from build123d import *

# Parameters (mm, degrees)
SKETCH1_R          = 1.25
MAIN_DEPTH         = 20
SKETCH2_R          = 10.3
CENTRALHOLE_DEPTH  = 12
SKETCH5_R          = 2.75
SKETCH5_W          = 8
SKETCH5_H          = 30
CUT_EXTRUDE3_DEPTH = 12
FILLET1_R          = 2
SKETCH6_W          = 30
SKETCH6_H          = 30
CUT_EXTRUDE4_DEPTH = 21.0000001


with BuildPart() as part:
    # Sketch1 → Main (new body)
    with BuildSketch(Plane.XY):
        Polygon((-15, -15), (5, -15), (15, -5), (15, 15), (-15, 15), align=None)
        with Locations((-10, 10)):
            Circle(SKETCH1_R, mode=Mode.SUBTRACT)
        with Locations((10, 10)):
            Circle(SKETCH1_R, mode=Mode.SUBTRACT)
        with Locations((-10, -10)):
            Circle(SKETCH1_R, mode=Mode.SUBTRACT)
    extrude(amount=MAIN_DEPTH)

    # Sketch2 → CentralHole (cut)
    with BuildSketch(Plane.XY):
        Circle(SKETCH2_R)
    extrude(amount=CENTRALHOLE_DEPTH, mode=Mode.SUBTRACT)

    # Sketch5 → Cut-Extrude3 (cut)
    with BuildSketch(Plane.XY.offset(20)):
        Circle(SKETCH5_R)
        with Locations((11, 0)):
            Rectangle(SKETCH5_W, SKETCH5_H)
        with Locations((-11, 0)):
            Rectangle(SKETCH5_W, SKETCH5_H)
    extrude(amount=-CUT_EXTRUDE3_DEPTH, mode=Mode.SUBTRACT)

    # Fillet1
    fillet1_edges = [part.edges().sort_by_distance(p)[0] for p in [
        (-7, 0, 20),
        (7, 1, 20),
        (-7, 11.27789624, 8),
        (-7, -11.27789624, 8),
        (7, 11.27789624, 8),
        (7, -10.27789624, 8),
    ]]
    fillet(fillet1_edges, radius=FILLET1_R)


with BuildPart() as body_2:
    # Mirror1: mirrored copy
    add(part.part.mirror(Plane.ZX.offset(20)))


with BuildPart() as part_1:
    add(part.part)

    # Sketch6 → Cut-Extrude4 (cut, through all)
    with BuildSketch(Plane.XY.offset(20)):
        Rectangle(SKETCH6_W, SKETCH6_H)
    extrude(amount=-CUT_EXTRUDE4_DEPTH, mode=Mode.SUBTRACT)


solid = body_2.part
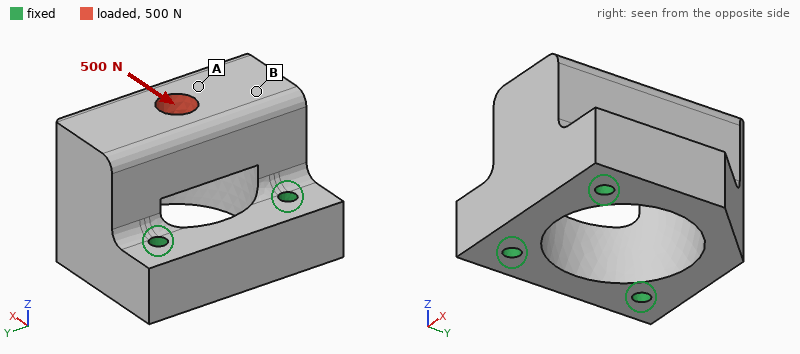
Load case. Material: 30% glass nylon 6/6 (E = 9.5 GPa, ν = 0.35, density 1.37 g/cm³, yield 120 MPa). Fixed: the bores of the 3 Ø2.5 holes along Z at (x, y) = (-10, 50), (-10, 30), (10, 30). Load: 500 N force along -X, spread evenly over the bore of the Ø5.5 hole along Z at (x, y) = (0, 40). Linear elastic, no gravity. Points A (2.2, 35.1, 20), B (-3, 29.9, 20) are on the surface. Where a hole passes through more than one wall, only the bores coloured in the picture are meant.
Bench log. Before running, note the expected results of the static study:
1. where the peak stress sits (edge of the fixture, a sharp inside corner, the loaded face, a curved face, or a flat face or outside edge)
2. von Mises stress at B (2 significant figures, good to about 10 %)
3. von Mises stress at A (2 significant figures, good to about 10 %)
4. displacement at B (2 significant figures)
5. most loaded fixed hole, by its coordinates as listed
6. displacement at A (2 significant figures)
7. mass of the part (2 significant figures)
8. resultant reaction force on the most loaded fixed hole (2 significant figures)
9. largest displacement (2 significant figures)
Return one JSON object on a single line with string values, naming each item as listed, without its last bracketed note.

{"where the peak stress sits": "edge of the fixture", "von Mises stress at B": "4.1 MPa", "von Mises stress at A": "8.5 MPa", "displacement at B": "32 µm", "most loaded fixed hole, by its coordinates as listed": "(10, 30)", "displacement at A": "42 µm", "mass of the part": "11 g", "resultant reaction force on the most loaded fixed hole": "290 N", "largest displacement": "59 µm"}
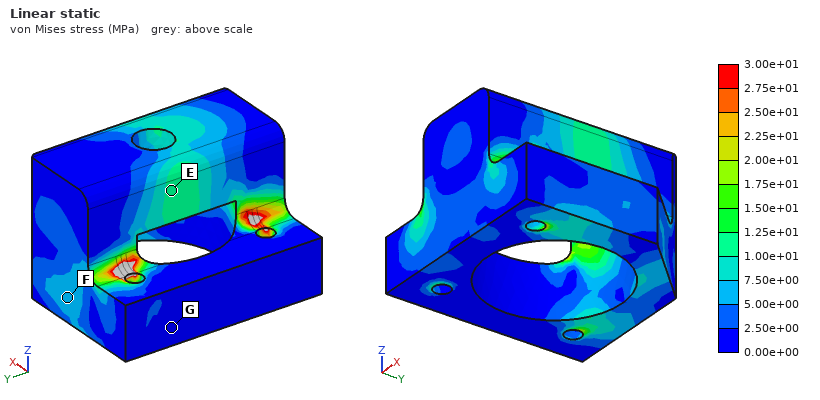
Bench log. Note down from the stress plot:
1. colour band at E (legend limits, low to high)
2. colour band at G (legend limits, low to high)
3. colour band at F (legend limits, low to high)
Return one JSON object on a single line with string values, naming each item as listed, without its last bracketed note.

{"colour band at E": "1.00e+01 to 1.25e+01 MPa", "colour band at G": "0.00e+00 to 2.50e+00 MPa", "colour band at F": "5.00e+00 to 7.50e+00 MPa"}
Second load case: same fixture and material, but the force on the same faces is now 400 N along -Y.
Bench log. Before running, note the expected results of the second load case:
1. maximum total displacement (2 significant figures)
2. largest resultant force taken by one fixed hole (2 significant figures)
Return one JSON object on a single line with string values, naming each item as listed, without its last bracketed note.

{"maximum total displacement": "42 µm", "largest resultant force taken by one fixed hole": "170 N"}
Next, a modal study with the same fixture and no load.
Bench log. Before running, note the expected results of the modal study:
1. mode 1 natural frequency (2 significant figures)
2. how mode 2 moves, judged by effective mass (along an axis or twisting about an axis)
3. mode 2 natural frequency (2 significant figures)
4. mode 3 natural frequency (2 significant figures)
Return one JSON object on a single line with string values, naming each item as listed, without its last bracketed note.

{"mode 1 natural frequency": "6600 Hz", "how mode 2 moves, judged by effective mass": "along Y", "mode 2 natural frequency": "8900 Hz", "mode 3 natural frequency": "13 kHz"}
